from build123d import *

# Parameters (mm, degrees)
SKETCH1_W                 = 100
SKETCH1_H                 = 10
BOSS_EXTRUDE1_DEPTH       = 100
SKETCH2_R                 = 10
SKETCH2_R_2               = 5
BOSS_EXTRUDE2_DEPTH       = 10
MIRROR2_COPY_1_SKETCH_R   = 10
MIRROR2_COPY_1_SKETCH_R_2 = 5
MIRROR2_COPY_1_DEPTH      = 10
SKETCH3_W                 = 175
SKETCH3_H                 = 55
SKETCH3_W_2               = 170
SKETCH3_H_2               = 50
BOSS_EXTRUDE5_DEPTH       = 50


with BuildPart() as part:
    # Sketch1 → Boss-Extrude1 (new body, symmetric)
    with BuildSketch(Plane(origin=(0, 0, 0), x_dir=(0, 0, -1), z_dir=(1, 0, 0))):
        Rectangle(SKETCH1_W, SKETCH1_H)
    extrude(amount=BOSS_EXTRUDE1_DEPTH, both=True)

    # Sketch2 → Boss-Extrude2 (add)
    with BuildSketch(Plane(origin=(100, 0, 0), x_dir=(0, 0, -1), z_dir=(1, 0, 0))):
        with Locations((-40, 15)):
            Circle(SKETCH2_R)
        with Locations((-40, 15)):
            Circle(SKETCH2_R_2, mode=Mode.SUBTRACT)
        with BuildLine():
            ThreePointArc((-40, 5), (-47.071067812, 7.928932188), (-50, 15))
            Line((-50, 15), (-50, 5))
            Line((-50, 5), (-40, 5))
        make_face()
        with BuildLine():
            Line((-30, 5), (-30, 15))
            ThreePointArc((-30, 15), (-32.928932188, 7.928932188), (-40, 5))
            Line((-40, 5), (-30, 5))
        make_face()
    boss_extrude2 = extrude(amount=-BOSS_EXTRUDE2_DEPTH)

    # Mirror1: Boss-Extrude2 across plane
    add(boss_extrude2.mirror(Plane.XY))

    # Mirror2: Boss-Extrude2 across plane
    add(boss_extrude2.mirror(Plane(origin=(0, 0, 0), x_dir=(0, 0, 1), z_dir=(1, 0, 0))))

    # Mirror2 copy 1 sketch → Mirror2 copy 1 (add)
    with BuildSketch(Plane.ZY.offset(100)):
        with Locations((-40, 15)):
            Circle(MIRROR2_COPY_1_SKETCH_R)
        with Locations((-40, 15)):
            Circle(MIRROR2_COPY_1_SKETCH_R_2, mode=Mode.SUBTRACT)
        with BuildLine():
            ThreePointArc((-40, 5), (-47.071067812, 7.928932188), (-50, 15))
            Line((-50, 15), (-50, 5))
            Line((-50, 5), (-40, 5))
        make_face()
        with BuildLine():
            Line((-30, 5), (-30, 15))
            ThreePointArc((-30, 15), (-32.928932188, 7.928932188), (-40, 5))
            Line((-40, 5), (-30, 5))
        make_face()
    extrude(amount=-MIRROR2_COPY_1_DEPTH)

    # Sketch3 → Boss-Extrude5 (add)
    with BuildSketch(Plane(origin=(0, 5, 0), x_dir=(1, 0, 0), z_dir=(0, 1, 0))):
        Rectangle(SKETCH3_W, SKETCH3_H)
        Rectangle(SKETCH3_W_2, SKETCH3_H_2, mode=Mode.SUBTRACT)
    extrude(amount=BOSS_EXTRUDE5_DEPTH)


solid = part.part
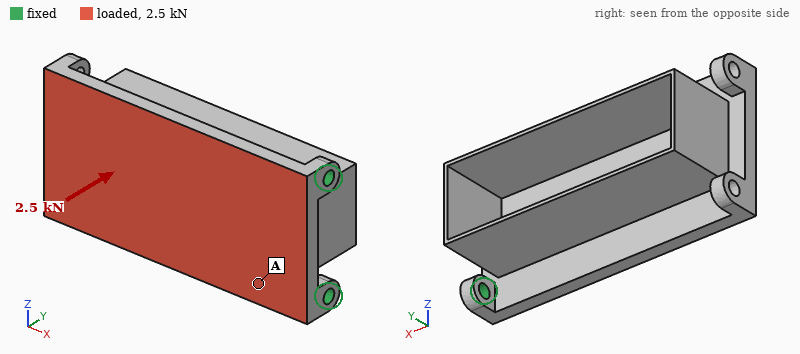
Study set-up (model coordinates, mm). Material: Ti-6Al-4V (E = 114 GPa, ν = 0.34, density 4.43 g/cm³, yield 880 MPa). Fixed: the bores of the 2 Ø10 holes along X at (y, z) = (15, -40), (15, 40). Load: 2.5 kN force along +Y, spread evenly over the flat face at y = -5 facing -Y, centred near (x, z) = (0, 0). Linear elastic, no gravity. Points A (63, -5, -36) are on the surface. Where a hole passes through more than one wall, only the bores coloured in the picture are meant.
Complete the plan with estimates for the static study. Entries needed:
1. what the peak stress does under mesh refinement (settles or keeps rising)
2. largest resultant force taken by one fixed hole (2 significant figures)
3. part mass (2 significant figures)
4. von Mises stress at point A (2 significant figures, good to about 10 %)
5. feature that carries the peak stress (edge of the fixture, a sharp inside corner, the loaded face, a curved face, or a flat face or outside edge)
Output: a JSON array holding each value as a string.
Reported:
["keeps rising", "1.3 kN", "1.2 kg", "38 MPa", "edge of the fixture"]
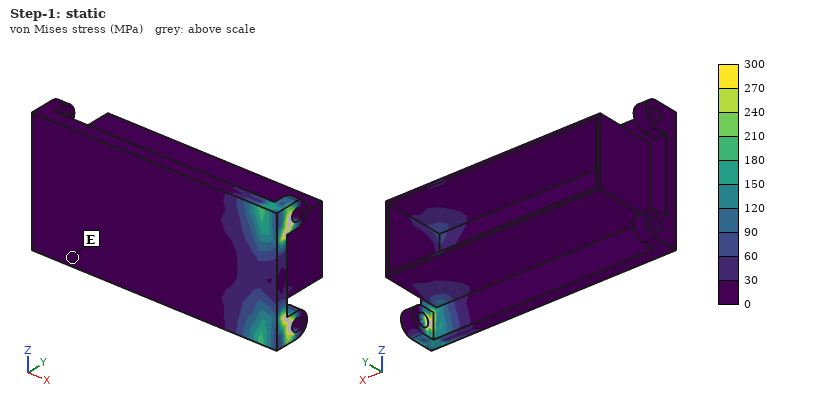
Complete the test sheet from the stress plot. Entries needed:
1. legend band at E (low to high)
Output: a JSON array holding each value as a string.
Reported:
["0 to 30 MPa"]
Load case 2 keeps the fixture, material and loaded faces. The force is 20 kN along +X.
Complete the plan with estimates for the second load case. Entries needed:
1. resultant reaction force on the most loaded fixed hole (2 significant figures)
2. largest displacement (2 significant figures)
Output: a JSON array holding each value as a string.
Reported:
["10 kN", "1.9 mm"]
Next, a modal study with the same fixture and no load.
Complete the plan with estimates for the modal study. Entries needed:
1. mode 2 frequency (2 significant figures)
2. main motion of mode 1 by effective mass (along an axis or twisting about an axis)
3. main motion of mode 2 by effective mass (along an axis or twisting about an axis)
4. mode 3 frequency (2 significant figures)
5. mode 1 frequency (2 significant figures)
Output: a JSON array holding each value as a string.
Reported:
["620 Hz", "along Y", "along Z", "1100 Hz", "180 Hz"]
